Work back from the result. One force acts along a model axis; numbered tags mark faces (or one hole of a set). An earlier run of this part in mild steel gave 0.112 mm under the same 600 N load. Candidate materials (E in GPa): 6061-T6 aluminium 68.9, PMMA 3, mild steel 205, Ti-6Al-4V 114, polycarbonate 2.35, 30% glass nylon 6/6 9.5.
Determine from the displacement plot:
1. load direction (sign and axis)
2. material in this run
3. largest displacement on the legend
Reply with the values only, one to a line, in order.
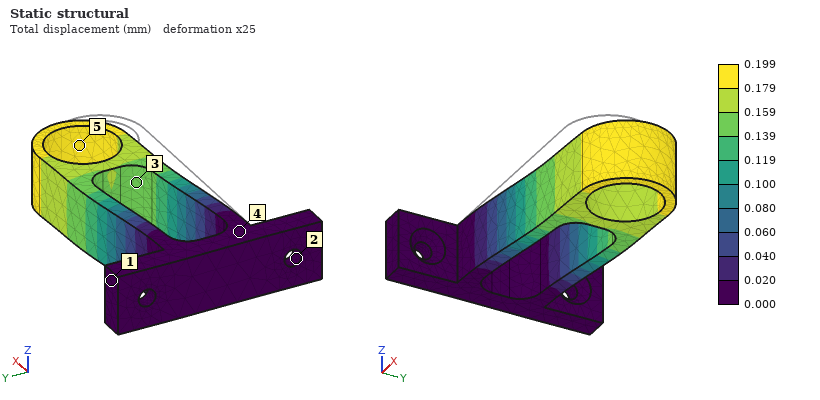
+Y
Ti-6Al-4V
0.199 mm
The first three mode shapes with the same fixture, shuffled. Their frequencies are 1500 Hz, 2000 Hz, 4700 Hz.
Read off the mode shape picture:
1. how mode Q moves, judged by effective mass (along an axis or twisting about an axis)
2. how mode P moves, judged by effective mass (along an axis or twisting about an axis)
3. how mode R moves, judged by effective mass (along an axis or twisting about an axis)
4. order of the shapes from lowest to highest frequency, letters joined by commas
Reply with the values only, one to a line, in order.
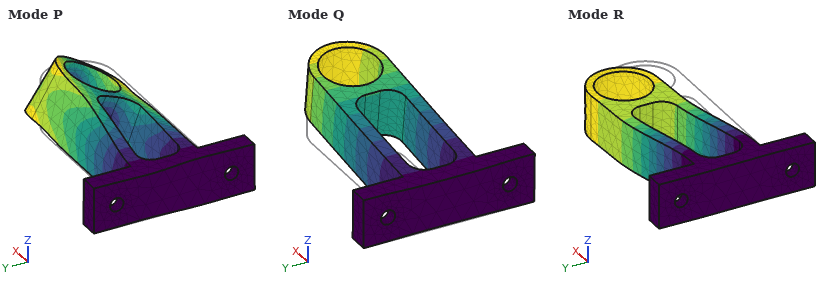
along Z
twisting about X
along Y
Q, R, P
